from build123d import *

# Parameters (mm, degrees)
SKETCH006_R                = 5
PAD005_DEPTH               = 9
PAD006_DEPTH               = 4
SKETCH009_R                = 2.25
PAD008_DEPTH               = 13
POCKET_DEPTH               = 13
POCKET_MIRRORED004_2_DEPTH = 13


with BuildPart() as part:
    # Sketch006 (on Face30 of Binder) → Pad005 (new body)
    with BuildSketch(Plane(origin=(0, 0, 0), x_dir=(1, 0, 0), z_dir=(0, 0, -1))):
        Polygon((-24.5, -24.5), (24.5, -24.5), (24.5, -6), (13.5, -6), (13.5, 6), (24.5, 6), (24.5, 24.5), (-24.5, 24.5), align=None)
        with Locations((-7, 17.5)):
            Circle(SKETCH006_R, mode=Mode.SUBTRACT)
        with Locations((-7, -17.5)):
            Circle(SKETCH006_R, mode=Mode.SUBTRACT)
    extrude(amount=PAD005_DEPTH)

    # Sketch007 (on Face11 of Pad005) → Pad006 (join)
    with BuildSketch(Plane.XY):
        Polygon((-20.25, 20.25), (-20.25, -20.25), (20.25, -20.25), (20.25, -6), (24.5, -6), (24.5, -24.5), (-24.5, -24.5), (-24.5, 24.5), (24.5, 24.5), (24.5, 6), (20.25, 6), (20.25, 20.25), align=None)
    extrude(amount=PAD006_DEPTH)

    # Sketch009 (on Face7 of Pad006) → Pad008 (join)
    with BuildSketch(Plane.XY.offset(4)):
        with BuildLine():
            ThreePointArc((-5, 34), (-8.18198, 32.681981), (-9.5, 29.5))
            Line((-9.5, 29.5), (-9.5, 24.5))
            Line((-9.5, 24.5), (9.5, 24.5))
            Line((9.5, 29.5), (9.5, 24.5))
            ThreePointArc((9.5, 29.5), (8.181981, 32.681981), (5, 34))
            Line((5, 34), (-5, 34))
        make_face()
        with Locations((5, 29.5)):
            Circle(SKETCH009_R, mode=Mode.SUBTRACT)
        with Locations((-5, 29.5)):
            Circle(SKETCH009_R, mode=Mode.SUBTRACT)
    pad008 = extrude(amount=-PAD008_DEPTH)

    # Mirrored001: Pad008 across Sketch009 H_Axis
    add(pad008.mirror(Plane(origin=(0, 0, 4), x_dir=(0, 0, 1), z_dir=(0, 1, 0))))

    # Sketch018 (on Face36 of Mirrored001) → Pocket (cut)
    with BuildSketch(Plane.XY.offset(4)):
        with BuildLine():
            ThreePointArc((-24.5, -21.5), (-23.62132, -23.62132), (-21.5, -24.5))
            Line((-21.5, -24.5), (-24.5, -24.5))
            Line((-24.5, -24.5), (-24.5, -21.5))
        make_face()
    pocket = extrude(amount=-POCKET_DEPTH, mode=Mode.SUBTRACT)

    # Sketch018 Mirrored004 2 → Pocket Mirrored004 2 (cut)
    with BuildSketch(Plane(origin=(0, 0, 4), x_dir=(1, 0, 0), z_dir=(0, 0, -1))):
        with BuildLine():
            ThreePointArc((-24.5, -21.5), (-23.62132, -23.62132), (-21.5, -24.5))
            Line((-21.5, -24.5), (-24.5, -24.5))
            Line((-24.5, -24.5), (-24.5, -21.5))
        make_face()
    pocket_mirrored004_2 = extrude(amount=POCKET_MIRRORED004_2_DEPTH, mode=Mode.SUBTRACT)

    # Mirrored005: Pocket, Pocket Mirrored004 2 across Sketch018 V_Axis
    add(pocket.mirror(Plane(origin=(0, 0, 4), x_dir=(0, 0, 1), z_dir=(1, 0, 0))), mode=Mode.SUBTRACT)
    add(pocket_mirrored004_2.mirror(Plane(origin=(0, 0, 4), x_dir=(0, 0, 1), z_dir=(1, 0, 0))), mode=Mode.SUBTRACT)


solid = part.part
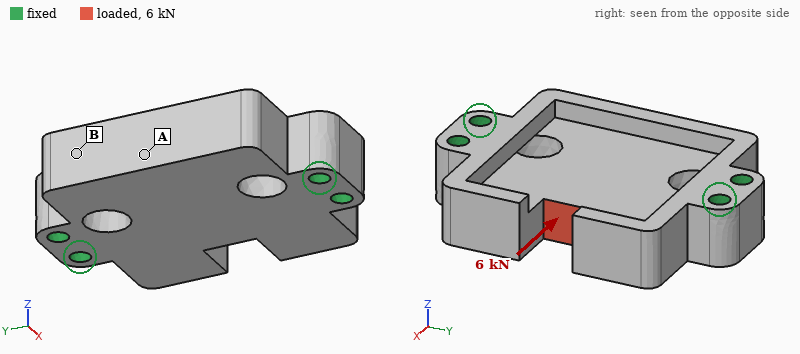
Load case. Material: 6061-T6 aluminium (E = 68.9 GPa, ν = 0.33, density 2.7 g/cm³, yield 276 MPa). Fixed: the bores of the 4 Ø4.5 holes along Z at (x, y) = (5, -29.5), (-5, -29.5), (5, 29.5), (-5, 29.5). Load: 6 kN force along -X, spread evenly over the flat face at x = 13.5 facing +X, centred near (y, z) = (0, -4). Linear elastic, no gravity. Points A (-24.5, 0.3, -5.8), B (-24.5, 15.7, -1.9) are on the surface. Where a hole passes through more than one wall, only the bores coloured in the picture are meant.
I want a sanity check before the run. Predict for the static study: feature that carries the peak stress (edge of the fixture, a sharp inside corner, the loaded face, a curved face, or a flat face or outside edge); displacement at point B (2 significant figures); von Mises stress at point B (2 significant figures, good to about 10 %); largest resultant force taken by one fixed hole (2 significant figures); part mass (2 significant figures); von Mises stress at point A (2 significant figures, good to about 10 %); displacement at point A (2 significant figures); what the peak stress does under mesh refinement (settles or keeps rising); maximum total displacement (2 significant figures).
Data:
edge of the fixture
13 µm
10 MPa
2.4 kN
69 g
25 MPa
17 µm
keeps rising
29 µm
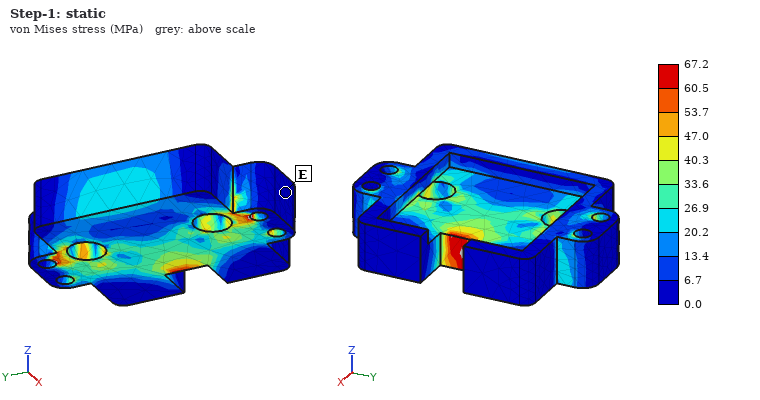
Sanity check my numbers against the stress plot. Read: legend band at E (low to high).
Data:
0.0 to 6.7 MPa
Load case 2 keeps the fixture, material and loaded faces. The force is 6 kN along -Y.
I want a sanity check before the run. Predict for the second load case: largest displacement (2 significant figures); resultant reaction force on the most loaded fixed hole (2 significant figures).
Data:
16 µm
2.1 kN
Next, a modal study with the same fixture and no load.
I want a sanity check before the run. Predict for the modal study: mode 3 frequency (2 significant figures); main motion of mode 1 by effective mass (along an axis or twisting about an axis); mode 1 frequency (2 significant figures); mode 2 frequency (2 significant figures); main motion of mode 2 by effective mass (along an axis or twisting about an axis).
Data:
14 kHz
along Z
8300 Hz
10 kHz
along Z
